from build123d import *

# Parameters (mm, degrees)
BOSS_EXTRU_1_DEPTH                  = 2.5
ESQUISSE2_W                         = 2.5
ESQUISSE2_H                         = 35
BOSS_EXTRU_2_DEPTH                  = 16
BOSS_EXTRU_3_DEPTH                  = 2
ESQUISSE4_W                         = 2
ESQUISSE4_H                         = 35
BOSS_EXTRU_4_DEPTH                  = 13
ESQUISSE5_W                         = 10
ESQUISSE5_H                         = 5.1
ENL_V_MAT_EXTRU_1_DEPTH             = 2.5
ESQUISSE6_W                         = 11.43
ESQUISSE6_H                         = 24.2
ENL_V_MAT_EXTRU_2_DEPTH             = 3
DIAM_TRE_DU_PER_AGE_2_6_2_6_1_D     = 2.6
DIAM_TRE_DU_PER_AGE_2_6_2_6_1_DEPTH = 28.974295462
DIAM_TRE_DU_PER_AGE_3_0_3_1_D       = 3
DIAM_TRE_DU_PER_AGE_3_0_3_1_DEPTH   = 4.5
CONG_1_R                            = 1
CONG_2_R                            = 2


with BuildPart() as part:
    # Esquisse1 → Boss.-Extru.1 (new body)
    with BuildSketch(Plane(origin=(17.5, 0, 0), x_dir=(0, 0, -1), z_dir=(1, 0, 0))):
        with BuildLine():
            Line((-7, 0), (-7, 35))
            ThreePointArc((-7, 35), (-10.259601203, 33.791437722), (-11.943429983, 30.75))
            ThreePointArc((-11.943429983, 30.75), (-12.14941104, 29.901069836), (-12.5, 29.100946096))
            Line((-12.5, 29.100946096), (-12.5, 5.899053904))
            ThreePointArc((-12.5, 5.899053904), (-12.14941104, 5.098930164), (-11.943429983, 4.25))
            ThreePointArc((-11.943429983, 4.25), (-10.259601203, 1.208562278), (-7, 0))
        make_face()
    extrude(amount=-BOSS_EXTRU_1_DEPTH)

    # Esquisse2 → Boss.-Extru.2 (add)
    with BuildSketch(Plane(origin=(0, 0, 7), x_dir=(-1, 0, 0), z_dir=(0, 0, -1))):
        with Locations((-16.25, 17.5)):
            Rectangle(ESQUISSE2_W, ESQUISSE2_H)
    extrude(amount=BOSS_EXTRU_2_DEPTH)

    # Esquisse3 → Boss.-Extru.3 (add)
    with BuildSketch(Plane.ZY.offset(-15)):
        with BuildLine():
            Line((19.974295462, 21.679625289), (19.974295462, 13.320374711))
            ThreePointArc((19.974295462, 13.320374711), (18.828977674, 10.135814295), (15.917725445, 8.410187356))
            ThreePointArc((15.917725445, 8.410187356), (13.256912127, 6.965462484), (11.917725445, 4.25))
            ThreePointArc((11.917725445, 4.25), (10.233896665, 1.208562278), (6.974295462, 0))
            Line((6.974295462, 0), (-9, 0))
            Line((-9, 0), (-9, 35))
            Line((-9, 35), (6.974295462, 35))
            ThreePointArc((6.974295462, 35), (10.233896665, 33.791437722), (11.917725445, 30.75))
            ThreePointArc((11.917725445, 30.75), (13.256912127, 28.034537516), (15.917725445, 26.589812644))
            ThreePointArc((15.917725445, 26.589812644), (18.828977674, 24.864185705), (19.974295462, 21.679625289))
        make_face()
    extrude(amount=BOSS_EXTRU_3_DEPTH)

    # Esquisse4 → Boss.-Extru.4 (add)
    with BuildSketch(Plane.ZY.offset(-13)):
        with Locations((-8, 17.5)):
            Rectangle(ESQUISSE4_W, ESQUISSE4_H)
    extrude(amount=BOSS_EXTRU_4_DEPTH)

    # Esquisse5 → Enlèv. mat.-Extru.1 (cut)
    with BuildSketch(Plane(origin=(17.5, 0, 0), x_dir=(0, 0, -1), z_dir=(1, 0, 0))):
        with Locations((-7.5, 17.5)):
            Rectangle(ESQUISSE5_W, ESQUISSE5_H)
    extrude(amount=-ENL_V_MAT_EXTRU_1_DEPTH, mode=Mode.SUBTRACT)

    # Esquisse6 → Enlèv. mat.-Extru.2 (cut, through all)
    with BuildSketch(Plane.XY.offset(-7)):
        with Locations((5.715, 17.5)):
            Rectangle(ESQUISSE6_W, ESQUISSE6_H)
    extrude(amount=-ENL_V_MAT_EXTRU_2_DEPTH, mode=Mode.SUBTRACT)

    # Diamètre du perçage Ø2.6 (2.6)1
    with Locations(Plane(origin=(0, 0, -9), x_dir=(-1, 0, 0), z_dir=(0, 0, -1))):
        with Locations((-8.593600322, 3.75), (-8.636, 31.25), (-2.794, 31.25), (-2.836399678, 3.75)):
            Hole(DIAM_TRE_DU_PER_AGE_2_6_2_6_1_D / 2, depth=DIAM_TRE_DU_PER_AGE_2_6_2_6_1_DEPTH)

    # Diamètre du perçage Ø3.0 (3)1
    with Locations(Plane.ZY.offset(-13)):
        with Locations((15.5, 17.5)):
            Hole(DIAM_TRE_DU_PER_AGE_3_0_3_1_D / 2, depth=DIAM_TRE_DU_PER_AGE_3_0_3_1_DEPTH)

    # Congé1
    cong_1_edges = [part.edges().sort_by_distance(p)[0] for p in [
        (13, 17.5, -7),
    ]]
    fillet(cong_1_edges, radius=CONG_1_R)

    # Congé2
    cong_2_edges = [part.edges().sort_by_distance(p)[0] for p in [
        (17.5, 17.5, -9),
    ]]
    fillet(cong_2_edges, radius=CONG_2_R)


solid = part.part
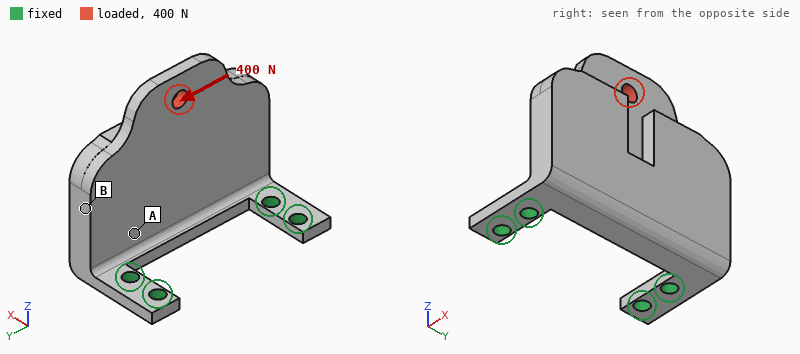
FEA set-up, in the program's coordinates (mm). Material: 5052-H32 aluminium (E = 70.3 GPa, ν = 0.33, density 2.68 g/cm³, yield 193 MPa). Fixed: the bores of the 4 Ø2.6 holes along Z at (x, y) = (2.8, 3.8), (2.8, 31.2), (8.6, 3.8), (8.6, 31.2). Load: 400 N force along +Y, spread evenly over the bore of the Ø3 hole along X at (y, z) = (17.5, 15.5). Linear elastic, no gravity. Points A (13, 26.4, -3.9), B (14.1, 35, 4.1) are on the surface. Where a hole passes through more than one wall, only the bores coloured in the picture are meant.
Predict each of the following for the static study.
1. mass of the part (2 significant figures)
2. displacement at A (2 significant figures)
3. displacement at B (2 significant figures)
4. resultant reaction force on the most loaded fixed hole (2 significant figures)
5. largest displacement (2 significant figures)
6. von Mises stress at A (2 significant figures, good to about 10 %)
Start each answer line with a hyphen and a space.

- 10.0 g
- 15 µm
- 38 µm
- 400 N
- 52 µm
- 32 MPa
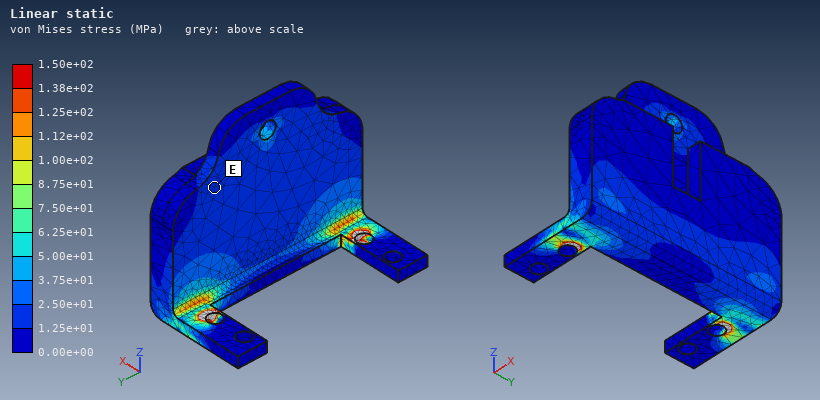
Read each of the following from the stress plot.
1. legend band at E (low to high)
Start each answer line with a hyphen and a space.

- 1.25e+01 to 2.50e+01 MPa
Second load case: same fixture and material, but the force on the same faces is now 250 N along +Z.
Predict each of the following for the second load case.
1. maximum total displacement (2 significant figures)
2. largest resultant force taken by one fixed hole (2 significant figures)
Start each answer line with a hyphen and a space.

- 0.13 mm
- 130 N
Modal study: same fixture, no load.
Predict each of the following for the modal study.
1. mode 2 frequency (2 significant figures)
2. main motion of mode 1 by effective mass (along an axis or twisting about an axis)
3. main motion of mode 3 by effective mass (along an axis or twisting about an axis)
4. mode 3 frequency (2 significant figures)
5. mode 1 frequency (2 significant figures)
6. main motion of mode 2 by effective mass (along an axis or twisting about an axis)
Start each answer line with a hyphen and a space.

- 7200 Hz
- along X
- along Z
- 10 kHz
- 1400 Hz
- along Y
